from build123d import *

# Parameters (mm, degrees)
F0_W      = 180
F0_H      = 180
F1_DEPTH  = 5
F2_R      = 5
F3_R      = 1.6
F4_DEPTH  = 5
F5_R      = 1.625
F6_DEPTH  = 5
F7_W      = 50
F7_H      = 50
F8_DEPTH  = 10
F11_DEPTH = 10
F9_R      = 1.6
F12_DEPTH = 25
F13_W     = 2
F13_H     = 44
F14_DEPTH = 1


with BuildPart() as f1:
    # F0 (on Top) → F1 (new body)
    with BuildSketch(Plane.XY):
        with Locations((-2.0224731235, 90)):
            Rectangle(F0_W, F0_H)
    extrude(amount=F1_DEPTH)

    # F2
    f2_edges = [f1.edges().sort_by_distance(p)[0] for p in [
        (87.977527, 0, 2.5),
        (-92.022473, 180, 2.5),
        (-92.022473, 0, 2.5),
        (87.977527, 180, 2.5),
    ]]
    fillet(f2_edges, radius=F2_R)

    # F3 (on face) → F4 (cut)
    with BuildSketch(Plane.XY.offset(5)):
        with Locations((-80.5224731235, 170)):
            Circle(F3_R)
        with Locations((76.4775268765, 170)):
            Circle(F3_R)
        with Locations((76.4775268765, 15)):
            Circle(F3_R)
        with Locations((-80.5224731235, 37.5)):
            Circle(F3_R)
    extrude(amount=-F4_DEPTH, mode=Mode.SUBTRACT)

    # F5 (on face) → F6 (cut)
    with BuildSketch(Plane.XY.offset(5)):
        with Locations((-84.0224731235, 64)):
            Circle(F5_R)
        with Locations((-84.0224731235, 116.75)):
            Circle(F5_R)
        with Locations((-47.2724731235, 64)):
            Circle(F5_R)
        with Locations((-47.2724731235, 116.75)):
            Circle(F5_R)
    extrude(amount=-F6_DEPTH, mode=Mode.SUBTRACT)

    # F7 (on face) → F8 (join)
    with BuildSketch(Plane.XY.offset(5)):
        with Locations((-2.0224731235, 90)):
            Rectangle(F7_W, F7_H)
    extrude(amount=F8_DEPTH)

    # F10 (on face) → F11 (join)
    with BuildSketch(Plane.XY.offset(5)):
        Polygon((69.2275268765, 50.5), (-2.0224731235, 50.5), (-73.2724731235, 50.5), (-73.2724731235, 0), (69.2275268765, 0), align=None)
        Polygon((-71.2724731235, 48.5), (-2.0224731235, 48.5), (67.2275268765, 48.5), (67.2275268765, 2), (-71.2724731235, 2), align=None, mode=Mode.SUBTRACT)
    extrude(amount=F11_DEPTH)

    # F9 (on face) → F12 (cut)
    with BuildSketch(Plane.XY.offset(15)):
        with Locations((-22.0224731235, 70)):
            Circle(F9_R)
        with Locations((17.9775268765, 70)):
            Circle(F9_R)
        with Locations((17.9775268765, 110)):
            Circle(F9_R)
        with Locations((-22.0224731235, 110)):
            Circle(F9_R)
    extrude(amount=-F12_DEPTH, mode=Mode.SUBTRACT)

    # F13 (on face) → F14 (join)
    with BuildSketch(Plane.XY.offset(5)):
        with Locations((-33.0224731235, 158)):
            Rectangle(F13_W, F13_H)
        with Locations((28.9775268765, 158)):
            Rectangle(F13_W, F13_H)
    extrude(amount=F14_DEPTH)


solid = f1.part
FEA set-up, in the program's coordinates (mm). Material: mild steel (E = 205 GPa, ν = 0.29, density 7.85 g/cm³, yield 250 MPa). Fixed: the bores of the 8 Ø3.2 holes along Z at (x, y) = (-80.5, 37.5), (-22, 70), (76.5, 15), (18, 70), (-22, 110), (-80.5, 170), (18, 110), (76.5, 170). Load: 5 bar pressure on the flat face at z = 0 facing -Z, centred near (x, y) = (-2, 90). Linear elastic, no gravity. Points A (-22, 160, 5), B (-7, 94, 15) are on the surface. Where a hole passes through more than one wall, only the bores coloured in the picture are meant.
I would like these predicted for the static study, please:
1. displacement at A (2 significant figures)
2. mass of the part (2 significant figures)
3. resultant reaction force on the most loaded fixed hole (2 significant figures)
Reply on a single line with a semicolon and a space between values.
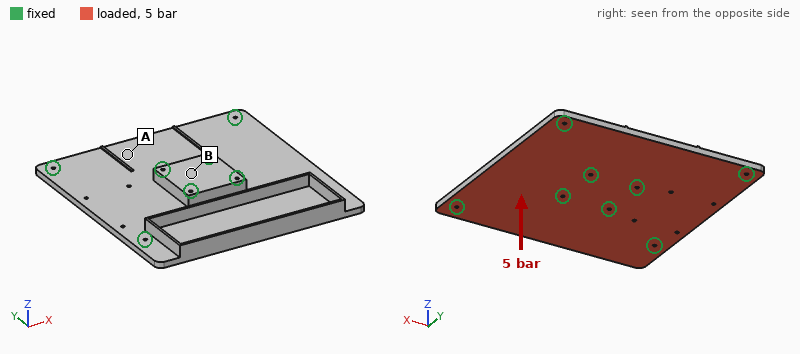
0.12 mm; 1.5 kg; 2.5 kN
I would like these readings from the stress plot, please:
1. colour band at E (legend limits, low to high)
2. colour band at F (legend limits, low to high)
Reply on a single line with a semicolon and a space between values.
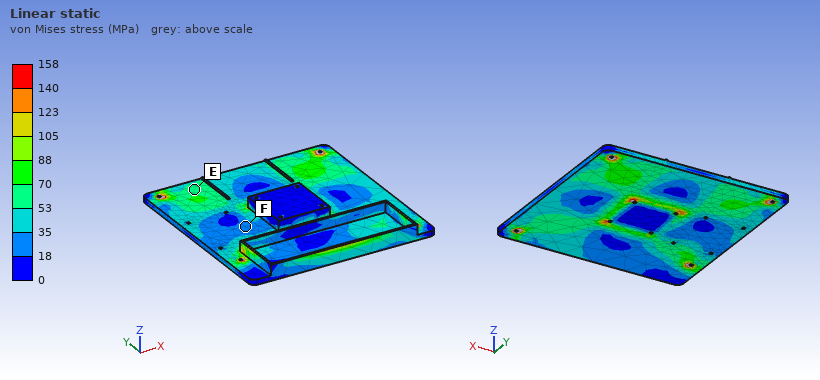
53 to 70 MPa; 18 to 35 MPa
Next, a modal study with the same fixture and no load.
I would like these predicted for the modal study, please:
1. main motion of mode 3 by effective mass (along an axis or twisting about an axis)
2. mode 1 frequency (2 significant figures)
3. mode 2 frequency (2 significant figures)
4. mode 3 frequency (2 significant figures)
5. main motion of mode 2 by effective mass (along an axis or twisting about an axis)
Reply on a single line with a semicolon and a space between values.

along Z; 1500 Hz; 1600 Hz; 1800 Hz; twisting about X
